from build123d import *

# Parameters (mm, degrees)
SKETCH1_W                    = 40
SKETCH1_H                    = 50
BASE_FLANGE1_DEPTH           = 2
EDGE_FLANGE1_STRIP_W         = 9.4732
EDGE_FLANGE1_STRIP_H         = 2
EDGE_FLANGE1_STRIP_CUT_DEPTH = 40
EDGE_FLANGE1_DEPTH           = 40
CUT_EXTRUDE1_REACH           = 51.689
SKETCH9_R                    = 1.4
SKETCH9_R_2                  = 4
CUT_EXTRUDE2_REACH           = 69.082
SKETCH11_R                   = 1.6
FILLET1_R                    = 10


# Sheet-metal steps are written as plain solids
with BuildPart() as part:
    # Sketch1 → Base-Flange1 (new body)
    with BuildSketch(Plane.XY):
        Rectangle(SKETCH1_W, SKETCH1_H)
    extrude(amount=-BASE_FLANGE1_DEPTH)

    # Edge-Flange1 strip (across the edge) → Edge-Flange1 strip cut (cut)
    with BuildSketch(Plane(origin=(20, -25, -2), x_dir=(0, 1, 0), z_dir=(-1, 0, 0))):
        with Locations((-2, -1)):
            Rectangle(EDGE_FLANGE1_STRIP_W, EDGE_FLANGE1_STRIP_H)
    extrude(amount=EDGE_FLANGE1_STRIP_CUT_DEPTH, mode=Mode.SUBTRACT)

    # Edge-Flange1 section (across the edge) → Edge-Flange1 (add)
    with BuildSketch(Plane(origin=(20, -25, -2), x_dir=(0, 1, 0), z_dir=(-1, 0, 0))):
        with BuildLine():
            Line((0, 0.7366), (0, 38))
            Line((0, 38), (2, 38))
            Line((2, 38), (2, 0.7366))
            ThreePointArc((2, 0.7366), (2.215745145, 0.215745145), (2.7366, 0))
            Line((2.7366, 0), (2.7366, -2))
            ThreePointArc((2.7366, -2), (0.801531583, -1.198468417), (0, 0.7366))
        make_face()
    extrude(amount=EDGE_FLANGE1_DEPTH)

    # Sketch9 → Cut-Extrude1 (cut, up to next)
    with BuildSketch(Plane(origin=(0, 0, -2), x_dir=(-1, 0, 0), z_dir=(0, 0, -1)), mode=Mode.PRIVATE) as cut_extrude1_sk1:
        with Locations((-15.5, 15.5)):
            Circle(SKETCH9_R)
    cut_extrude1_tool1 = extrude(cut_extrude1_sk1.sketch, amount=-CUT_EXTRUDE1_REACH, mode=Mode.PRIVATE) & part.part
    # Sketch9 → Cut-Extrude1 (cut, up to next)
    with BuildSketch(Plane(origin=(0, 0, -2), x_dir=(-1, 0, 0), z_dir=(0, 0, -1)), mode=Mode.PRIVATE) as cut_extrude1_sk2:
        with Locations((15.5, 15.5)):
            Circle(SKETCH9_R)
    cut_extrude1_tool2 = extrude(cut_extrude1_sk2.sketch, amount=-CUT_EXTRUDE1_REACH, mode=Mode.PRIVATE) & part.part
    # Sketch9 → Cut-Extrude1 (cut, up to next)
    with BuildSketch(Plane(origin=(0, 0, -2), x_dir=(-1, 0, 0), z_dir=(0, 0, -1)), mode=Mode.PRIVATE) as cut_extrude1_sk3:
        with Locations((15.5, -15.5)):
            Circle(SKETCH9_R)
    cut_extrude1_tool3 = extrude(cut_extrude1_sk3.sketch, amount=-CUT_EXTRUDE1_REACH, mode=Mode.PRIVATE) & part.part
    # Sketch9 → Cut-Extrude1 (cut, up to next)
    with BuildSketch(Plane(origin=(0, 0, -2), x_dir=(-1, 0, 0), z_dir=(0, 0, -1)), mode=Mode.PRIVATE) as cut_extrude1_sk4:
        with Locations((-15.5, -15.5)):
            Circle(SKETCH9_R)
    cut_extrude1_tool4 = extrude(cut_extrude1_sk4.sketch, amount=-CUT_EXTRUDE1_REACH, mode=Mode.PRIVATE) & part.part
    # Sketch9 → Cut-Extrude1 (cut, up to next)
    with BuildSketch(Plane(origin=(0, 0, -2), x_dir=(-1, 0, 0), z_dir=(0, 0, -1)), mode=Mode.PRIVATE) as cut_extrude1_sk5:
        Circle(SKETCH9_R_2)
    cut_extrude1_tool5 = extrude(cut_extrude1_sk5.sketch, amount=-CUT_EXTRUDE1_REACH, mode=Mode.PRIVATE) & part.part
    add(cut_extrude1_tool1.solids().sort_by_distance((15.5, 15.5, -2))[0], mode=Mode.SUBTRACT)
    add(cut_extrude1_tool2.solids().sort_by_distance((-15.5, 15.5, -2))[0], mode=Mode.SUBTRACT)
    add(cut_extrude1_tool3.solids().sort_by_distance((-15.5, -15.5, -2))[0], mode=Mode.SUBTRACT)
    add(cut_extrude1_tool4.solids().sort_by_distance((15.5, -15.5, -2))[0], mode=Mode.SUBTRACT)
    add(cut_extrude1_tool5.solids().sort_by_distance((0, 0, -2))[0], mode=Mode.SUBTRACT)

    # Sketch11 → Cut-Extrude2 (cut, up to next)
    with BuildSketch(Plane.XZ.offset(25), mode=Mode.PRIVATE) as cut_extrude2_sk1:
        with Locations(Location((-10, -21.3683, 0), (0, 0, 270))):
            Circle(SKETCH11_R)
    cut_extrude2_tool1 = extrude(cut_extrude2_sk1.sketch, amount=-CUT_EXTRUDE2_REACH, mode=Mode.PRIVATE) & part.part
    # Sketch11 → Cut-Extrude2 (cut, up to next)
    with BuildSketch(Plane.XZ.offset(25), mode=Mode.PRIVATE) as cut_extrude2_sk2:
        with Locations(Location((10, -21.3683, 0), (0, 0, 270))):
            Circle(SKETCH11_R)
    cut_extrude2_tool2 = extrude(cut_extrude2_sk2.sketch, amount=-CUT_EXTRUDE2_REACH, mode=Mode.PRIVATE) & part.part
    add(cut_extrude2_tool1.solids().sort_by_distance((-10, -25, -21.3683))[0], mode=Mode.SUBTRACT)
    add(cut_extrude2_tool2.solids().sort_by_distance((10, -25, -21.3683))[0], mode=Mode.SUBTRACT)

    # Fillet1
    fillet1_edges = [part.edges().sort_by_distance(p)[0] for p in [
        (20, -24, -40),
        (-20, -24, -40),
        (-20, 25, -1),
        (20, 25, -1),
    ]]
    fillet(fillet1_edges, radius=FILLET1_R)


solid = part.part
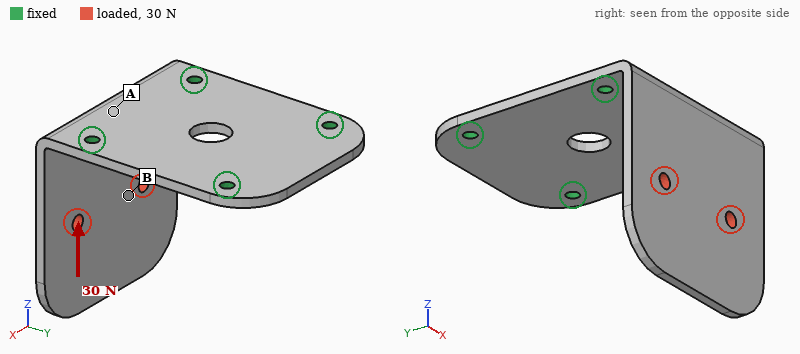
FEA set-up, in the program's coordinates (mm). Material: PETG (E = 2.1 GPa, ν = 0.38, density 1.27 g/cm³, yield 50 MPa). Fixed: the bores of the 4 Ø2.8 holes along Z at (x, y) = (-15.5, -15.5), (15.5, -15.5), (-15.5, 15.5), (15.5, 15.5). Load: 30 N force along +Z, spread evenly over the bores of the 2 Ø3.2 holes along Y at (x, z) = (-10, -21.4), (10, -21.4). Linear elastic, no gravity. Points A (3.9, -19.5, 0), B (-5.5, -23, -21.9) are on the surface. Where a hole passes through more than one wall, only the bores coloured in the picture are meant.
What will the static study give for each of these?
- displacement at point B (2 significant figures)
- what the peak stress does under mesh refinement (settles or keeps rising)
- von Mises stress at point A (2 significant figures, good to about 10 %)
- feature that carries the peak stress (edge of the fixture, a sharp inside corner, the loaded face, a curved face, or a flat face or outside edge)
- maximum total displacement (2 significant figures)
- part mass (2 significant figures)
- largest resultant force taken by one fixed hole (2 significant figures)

0.43 mm
keeps rising
2.4 MPa
edge of the fixture
0.79 mm
8.4 g
16 N
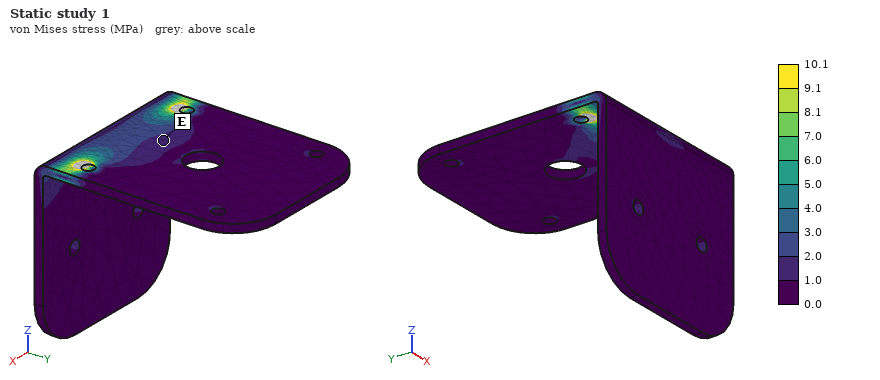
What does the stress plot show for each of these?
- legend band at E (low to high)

1.0 to 2.0 MPa
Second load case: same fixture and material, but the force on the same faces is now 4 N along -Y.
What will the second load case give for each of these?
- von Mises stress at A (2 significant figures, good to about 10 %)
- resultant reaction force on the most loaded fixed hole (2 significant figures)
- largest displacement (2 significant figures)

2.2 MPa
1.5 N
0.87 mm
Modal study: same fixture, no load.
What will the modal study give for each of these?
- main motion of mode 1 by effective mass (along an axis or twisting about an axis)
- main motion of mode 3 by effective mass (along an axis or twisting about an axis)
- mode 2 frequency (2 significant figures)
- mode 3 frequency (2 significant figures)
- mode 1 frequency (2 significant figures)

along Y
along X
600 Hz
980 Hz
220 Hz
